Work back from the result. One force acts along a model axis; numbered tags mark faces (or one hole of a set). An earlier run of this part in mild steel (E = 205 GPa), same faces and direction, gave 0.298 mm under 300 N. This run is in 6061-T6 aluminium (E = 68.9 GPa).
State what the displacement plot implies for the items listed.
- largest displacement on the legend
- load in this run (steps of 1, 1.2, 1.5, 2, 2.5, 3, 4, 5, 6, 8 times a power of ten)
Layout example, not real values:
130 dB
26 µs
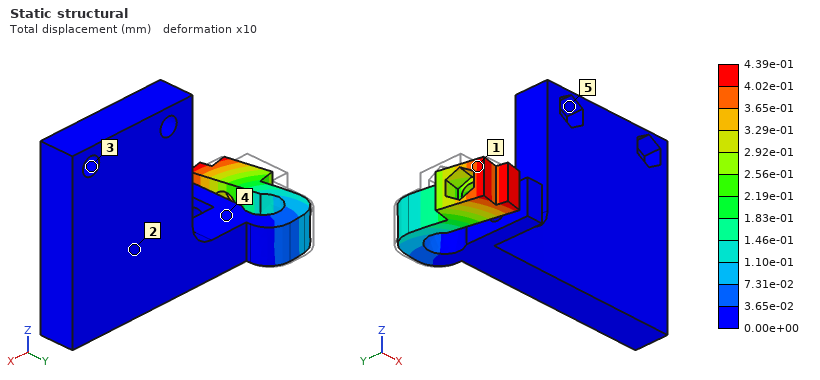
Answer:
4.39e-01 mm
150 N
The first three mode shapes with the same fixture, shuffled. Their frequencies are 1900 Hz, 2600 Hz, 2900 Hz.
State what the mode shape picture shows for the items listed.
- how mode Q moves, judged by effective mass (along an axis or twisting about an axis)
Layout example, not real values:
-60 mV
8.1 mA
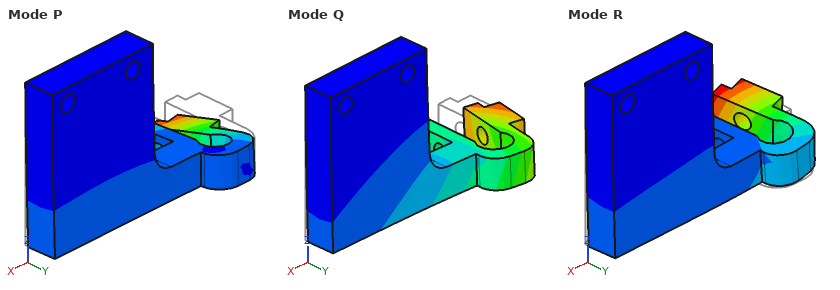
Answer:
along Y
